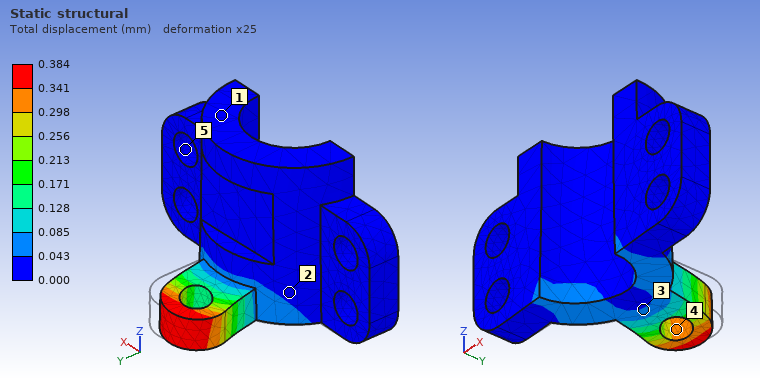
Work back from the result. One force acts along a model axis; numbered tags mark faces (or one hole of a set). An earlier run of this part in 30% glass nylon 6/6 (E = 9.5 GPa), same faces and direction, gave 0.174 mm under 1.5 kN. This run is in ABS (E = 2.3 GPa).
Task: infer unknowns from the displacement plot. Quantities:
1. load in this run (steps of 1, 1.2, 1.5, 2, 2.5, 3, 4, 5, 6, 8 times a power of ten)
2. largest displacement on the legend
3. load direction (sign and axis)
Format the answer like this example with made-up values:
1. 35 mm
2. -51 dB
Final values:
1. 800 N
2. 0.384 mm
3. -X
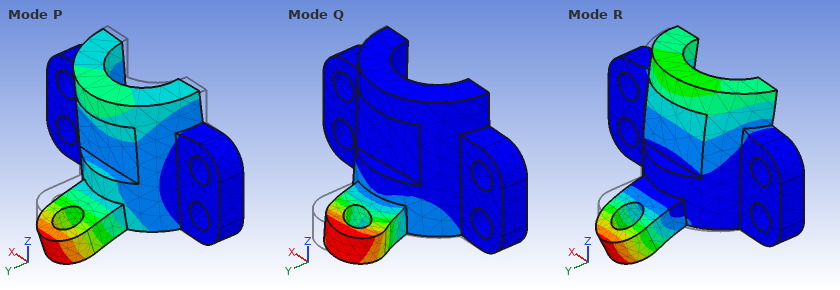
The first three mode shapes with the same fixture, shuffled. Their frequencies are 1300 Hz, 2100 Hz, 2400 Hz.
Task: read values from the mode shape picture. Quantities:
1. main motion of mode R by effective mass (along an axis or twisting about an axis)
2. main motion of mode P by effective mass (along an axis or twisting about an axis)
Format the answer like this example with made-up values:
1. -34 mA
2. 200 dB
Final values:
1. along Y
2. along Z
